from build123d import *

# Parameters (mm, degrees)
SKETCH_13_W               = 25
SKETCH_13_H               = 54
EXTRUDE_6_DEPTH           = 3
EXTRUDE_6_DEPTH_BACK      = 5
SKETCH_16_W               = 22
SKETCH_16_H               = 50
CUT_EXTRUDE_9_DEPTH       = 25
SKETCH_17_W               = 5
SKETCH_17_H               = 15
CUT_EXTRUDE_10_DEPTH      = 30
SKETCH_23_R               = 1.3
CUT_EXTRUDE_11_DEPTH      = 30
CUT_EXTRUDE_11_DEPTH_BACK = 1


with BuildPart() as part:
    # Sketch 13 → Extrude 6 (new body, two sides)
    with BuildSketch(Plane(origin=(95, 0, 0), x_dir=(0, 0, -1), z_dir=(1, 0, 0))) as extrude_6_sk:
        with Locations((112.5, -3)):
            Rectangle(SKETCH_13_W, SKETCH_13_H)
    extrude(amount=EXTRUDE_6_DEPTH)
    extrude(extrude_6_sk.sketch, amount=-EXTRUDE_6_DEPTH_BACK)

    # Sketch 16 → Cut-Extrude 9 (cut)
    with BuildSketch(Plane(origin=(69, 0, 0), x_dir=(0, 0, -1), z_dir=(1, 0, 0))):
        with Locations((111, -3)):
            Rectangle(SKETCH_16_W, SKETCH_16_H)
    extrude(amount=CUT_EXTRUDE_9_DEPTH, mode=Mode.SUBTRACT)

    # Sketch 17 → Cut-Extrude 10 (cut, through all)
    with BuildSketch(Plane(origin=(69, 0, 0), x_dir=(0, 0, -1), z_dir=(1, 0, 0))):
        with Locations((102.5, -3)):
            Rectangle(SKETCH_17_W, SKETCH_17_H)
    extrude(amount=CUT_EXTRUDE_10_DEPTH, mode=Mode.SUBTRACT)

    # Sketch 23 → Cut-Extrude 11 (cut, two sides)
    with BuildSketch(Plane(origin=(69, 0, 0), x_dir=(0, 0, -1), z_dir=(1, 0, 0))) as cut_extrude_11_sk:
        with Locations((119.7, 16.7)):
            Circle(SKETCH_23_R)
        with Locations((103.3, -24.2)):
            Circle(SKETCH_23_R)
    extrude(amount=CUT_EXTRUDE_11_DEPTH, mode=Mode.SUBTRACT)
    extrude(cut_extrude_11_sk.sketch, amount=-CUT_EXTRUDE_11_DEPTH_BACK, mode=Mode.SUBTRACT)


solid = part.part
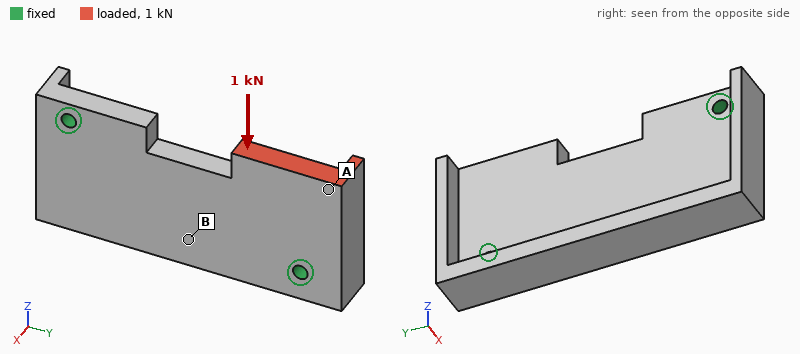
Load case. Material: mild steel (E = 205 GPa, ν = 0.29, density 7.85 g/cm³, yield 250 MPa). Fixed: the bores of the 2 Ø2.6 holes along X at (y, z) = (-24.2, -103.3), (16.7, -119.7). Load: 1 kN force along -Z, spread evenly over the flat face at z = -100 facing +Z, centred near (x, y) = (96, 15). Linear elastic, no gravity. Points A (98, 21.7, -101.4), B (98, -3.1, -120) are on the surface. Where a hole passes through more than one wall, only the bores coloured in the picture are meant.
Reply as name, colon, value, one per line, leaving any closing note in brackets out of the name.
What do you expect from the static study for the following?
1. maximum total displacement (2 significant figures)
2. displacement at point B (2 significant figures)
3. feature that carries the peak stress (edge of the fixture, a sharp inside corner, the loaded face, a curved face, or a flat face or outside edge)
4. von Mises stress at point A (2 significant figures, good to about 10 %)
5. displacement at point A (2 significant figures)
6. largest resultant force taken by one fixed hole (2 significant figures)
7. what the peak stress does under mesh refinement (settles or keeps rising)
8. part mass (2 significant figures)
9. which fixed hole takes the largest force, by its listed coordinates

maximum total displacement: 2.8 µm
displacement at point B: 0.69 µm
feature that carries the peak stress: edge of the fixture
von Mises stress at point A: 12 MPa
displacement at point A: 2.0 µm
largest resultant force taken by one fixed hole: 930 N
what the peak stress does under mesh refinement: keeps rising
part mass: 48 g
which fixed hole takes the largest force, by its listed coordinates: (16.7, -119.7)
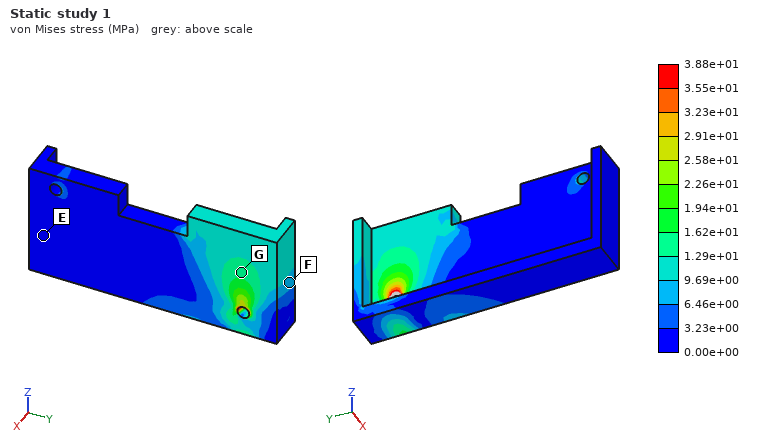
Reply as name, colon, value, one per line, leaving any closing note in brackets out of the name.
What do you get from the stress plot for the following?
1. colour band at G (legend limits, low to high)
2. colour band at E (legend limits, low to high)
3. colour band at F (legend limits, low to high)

colour band at G: 1.29e+01 to 1.62e+01 MPa
colour band at E: 0.00e+00 to 3.23e+00 MPa
colour band at F: 6.46e+00 to 9.69e+00 MPa
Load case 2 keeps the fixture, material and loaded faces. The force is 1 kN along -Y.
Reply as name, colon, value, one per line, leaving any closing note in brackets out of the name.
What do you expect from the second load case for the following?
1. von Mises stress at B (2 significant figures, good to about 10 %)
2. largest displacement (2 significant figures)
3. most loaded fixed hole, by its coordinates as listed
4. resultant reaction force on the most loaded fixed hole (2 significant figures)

von Mises stress at B: 17 MPa
largest displacement: 16 µm
most loaded fixed hole, by its coordinates as listed: (16.7, -119.7)
resultant reaction force on the most loaded fixed hole: 900 N
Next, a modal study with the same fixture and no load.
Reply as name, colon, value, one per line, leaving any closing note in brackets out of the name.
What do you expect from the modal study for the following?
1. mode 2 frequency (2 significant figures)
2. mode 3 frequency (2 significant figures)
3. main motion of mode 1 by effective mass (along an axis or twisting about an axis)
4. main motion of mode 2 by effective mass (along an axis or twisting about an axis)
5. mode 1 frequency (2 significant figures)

mode 2 frequency: 8100 Hz
mode 3 frequency: 12 kHz
main motion of mode 1 by effective mass: along X
main motion of mode 2 by effective mass: along X
mode 1 frequency: 6200 Hz
